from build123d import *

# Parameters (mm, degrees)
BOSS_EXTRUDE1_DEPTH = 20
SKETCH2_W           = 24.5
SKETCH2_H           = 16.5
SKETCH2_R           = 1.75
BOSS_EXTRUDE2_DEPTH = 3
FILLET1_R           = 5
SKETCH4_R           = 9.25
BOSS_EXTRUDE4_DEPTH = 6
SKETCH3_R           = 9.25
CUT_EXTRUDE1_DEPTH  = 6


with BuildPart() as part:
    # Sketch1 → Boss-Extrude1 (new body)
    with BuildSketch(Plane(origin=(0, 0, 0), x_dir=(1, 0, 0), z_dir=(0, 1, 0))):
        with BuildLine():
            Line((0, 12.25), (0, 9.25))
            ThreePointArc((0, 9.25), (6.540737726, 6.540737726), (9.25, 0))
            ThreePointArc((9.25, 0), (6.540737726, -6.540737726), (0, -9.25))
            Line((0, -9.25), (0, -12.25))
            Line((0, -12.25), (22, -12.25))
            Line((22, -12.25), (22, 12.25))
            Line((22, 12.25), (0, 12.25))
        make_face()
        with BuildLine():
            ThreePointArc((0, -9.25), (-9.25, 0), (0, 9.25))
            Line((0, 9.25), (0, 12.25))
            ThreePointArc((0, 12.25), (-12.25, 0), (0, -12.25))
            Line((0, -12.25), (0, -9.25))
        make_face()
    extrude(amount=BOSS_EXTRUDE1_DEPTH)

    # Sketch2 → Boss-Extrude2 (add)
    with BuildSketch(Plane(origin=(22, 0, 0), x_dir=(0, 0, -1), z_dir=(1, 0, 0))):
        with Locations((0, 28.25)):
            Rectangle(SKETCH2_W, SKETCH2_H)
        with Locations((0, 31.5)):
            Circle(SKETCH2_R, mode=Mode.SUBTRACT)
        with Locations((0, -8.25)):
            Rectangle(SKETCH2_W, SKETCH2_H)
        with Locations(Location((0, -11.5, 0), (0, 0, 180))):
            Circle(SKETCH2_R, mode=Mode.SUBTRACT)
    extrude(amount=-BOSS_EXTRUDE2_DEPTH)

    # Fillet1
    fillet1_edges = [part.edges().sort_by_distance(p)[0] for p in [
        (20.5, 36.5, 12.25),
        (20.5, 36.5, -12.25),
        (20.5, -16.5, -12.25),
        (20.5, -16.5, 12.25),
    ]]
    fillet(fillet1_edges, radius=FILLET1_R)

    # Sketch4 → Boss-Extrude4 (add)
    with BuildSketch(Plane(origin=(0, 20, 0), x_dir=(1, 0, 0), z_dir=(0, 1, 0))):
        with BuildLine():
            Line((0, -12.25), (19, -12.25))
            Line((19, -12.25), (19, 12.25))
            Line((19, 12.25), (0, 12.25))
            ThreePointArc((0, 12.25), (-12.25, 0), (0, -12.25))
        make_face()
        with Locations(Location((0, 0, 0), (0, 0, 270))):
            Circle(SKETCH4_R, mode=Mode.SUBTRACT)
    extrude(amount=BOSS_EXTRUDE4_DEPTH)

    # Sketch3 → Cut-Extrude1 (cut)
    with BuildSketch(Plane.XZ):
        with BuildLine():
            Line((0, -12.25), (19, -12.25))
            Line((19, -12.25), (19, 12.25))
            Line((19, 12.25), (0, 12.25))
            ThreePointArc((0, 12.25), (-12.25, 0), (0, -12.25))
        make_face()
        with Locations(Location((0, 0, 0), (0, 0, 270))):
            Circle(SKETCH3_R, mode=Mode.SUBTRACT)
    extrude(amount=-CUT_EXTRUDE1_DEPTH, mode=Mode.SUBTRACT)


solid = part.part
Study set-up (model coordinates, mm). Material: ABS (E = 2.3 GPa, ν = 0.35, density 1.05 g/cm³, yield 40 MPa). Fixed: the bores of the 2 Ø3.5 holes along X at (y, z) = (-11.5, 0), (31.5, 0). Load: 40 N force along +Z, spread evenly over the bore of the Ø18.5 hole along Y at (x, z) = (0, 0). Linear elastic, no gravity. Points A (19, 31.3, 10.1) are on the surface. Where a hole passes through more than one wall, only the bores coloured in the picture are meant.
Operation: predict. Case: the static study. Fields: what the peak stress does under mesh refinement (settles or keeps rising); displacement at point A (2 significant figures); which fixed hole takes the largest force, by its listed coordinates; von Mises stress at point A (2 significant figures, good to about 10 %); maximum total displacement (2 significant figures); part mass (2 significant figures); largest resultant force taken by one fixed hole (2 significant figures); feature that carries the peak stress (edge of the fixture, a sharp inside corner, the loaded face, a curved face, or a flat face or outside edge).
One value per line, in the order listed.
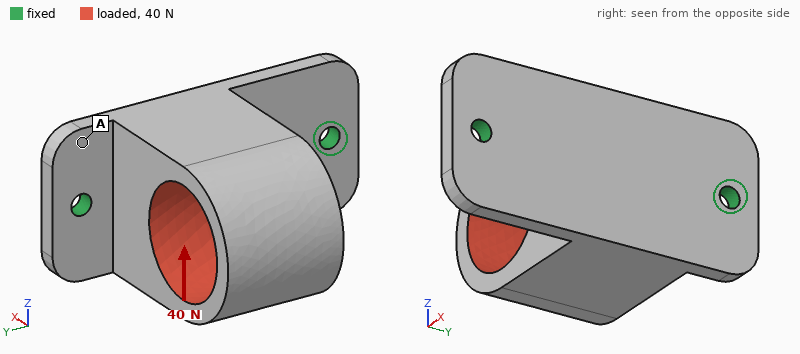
keeps rising
0.14 mm
(31.5, 0)
2.4 MPa
0.66 mm
13 g
27 N
edge of the fixture
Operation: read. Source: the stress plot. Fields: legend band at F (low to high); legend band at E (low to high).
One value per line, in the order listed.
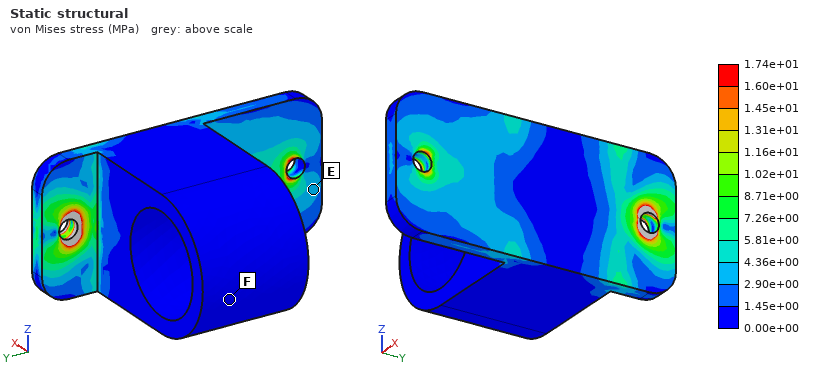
0.00e+00 to 1.45e+00 MPa
2.90e+00 to 4.36e+00 MPa
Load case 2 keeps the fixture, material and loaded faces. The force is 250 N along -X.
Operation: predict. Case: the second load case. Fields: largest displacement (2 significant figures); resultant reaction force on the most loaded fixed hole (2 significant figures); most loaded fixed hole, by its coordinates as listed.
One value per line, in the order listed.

0.61 mm
170 N
(31.5, 0)
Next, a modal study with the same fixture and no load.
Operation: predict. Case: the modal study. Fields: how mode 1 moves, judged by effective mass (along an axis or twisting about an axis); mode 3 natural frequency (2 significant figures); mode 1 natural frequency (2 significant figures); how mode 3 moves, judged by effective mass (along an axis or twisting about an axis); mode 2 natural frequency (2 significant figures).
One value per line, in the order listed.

along Z
2400 Hz
590 Hz
along X
1000 Hz
